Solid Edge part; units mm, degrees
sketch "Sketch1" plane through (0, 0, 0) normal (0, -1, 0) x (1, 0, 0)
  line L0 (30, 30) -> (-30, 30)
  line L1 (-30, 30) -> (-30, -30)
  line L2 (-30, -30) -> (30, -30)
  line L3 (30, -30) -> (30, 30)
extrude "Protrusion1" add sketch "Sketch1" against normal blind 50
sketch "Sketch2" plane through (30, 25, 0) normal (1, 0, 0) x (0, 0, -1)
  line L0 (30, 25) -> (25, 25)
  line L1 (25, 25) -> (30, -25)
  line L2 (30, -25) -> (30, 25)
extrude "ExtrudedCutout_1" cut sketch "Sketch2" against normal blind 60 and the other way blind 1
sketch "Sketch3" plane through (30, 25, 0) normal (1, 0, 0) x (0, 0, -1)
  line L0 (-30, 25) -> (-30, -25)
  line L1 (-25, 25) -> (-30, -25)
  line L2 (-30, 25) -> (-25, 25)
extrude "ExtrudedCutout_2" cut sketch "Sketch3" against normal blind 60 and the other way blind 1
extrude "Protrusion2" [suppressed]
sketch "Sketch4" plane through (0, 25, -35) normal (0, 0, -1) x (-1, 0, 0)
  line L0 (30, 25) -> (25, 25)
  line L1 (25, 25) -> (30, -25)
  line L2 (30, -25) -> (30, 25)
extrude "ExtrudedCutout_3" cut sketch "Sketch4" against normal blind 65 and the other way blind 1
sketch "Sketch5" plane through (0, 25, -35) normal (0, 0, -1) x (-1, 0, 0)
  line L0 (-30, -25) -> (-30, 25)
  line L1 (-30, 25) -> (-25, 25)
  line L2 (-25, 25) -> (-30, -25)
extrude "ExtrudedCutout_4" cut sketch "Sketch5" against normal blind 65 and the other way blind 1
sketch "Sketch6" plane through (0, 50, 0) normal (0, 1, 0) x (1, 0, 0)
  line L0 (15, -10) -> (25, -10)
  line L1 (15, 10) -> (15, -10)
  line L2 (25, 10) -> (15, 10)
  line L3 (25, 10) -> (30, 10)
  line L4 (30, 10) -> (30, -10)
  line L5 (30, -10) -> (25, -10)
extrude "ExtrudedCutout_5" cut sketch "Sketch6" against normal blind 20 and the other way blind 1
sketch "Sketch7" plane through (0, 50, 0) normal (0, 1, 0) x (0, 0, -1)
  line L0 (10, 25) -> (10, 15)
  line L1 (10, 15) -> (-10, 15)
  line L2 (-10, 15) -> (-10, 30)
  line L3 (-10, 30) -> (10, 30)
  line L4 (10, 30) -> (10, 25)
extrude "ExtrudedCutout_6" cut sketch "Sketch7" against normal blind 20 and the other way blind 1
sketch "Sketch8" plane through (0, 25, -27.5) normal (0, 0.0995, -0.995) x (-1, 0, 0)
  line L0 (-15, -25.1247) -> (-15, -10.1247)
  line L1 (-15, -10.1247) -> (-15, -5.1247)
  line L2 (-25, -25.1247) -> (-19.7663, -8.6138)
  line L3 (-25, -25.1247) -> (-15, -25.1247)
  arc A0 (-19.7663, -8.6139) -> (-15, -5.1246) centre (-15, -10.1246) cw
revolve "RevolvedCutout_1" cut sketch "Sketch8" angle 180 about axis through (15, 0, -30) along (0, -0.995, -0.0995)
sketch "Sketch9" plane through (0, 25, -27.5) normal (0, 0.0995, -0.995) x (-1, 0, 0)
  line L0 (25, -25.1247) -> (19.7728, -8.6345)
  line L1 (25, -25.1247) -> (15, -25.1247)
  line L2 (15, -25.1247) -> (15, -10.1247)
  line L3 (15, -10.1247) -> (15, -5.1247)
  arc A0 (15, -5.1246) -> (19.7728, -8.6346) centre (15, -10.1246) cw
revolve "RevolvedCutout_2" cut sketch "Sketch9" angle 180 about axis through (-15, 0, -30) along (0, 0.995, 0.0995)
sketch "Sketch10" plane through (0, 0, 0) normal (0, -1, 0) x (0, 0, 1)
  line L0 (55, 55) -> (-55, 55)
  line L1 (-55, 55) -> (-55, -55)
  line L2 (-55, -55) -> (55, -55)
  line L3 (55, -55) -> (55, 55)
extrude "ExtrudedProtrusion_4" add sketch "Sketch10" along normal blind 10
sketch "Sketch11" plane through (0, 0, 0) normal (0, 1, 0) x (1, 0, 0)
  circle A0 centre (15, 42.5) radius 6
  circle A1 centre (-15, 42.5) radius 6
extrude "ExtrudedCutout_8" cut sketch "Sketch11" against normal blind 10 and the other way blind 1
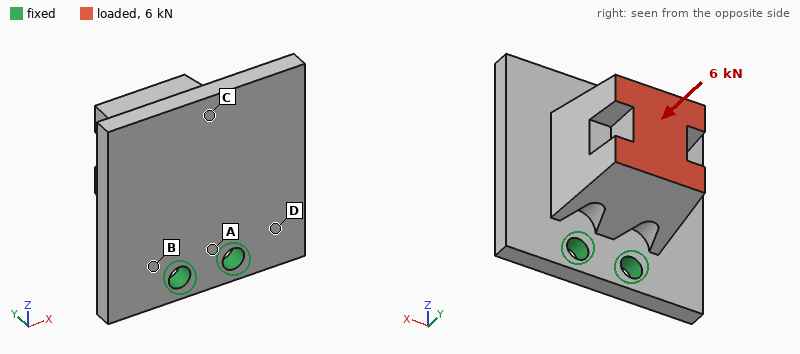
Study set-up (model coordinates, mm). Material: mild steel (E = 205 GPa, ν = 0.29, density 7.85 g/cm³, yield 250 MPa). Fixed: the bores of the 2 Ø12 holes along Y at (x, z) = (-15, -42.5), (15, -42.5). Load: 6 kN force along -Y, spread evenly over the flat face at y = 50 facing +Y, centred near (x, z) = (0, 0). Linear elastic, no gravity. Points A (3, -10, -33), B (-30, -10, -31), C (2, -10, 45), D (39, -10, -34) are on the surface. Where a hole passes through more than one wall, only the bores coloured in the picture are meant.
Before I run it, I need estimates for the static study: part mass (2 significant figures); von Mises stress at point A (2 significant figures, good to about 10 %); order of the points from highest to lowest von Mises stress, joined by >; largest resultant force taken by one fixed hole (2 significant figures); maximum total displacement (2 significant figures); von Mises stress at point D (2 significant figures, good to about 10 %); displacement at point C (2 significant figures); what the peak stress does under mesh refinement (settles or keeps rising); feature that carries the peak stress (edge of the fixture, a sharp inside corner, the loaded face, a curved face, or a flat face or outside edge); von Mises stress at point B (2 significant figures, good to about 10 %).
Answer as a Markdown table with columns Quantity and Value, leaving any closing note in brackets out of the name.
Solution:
| Quantity | Value |
|---|---|
| part mass | 2.0 kg |
| von Mises stress at point A | 110 MPa |
| order of the points from highest to lowest von Mises stress, joined by > | A > B > D > C |
| largest resultant force taken by one fixed hole | 3.0 kN |
| maximum total displacement | 0.21 mm |
| von Mises stress at point D | 56 MPa |
| displacement at point C | 0.18 mm |
| what the peak stress does under mesh refinement | keeps rising |
| feature that carries the peak stress | edge of the fixture |
| von Mises stress at point B | 80 MPa |
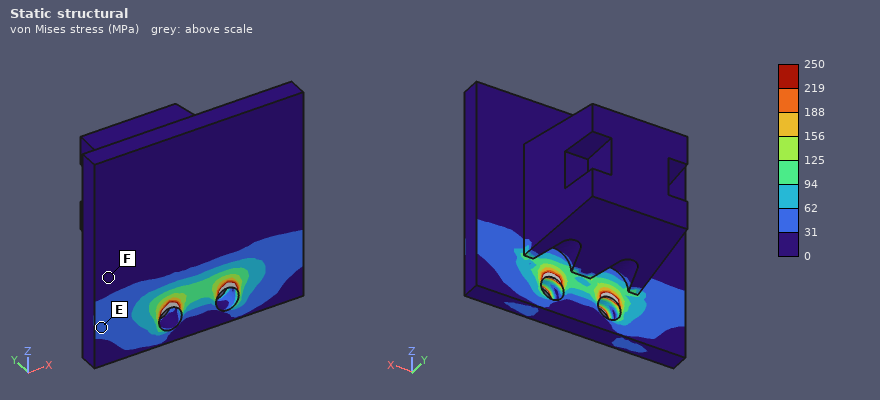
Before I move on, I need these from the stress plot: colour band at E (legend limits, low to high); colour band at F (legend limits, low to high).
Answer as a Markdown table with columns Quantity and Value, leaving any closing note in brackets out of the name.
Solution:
| Quantity | Value |
|---|---|
| colour band at E | 31 to 62 MPa |
| colour band at F | 0 to 31 MPa |
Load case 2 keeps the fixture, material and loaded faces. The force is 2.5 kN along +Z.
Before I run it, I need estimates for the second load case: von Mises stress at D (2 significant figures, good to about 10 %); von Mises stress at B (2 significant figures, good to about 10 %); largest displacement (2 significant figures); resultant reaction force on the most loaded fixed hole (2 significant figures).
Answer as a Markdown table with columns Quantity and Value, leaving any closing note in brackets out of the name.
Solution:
| Quantity | Value |
|---|---|
| von Mises stress at D | 43 MPa |
| von Mises stress at B | 60 MPa |
| largest displacement | 0.15 mm |
| resultant reaction force on the most loaded fixed hole | 1.3 kN |
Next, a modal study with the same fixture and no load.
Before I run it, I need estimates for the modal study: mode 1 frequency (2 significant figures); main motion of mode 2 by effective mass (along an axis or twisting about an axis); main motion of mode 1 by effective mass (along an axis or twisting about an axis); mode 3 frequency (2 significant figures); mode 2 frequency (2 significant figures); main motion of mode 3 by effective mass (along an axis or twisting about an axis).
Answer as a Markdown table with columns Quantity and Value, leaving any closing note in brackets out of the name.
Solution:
| Quantity | Value |
|---|---|
| mode 1 frequency | 680 Hz |
| main motion of mode 2 by effective mass | along X |
| main motion of mode 1 by effective mass | along Y |
| mode 3 frequency | 2800 Hz |
| mode 2 frequency | 2100 Hz |
| main motion of mode 3 by effective mass | along X |
